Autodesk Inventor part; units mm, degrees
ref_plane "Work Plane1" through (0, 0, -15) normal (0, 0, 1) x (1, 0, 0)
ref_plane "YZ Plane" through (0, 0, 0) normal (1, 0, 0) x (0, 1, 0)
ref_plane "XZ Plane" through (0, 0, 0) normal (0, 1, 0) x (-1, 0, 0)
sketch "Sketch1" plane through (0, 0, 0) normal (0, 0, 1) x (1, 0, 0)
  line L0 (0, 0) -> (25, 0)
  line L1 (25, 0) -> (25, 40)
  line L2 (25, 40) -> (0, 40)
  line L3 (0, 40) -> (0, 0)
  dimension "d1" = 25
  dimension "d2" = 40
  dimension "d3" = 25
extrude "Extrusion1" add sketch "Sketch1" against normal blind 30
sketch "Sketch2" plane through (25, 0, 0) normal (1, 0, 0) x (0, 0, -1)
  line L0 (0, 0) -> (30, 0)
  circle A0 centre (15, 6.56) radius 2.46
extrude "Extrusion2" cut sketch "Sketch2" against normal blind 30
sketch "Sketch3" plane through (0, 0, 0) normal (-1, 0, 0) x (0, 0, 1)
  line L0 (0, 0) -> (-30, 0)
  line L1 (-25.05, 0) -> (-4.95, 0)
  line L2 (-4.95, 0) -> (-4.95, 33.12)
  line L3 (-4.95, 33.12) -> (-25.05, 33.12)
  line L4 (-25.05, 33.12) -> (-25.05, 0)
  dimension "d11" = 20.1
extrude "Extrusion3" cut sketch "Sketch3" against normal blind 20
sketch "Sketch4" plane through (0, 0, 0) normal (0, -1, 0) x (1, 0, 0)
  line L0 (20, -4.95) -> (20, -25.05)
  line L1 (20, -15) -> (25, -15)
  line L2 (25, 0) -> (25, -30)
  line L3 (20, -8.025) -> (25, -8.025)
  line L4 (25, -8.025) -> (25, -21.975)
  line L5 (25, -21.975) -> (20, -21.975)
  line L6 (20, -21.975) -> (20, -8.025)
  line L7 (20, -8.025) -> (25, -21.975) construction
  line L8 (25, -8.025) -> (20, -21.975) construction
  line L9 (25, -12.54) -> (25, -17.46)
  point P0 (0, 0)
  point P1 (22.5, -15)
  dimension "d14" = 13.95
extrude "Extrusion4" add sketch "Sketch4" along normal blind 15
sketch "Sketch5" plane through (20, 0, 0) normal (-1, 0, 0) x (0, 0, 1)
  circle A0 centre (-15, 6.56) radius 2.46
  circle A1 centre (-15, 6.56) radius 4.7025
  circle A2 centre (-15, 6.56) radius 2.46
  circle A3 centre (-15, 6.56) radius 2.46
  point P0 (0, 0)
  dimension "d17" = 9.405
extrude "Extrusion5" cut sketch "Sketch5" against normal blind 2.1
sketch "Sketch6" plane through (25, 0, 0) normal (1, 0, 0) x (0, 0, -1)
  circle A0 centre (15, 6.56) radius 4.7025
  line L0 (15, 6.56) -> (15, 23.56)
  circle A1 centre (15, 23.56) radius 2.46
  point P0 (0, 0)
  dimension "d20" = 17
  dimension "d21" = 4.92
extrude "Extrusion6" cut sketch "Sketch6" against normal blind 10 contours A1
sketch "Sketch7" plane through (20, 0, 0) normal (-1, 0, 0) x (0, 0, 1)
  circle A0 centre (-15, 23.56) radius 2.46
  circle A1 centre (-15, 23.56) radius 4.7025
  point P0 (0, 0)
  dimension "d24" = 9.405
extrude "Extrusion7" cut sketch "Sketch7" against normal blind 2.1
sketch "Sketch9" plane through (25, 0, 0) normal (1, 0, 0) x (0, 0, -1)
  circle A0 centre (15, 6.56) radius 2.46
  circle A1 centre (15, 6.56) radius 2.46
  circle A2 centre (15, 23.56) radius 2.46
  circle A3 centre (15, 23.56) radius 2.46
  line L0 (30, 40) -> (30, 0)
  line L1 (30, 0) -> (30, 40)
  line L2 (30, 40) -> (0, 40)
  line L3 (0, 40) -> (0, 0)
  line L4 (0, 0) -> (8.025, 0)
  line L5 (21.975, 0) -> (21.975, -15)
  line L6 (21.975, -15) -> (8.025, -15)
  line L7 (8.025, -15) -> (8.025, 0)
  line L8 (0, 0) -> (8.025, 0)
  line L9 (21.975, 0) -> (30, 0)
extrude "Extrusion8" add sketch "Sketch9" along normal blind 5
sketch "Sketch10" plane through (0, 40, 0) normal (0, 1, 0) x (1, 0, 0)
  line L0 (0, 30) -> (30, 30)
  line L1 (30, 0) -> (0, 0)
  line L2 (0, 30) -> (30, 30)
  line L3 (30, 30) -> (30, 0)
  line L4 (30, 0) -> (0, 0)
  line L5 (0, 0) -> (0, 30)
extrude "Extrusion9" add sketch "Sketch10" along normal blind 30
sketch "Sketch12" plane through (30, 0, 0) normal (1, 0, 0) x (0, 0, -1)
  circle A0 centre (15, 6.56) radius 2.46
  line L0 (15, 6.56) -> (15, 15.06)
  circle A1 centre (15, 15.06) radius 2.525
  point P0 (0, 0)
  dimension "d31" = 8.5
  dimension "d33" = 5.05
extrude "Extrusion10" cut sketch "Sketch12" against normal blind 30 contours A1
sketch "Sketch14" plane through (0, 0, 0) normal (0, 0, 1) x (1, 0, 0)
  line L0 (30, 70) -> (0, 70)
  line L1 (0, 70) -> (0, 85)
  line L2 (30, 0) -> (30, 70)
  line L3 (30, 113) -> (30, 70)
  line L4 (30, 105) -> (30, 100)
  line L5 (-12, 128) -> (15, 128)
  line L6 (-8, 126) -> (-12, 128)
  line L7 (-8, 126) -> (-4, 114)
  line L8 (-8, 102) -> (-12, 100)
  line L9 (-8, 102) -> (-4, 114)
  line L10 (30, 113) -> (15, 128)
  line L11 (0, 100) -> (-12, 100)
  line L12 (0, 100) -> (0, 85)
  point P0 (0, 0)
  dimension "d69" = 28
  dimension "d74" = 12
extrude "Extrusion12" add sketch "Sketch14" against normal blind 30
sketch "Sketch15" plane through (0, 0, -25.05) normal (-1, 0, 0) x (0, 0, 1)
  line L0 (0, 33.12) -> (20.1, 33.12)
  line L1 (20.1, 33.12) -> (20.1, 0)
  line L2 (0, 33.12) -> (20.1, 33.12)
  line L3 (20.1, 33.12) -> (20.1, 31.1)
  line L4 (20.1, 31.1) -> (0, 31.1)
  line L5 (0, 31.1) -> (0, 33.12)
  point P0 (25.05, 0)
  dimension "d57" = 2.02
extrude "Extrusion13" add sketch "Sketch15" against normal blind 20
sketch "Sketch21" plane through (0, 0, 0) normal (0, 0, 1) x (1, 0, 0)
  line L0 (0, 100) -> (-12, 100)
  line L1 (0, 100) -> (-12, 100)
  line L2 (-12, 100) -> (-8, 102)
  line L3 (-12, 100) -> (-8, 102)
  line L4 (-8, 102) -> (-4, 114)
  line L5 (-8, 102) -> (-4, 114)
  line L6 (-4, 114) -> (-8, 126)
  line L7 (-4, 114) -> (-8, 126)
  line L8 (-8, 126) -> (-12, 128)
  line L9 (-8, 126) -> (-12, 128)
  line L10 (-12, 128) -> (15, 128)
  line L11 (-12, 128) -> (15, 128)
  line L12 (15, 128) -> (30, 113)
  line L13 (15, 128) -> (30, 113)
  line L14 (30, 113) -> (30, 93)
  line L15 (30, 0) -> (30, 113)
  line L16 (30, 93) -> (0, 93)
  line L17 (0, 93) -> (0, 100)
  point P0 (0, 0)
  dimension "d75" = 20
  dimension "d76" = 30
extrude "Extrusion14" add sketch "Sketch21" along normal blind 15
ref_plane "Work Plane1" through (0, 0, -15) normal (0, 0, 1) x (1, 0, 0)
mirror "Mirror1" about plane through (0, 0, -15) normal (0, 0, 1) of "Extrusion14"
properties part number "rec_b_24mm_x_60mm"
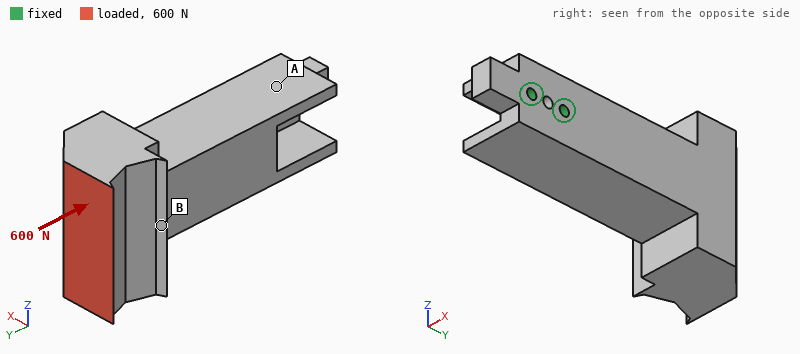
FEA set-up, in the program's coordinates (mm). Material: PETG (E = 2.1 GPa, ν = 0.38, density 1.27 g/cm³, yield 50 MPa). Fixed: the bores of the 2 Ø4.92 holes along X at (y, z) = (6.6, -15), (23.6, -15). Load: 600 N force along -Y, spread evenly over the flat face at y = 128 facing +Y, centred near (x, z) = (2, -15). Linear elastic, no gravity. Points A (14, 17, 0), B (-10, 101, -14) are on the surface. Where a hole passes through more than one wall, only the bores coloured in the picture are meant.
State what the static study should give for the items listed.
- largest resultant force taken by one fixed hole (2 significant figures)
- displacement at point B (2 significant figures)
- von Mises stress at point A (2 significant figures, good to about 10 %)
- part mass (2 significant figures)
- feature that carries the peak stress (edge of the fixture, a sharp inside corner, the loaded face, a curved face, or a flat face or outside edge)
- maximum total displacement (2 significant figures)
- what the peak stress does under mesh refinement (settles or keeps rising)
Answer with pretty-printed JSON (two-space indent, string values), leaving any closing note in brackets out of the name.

{
  "largest resultant force taken by one fixed hole": "670 N",
  "displacement at point B": "1.1 mm",
  "von Mises stress at point A": "4.3 MPa",
  "part mass": "180 g",
  "feature that carries the peak stress": "edge of the fixture",
  "maximum total displacement": "1.5 mm",
  "what the peak stress does under mesh refinement": "keeps rising"
}
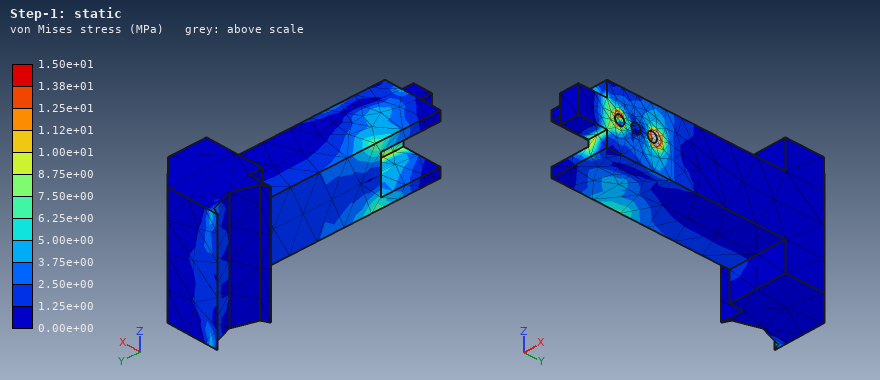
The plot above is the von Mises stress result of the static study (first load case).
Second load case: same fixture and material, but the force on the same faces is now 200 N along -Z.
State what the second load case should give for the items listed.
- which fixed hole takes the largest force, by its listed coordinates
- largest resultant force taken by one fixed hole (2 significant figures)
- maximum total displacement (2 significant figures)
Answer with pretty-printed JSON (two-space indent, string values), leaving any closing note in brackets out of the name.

{
  "which fixed hole takes the largest force, by its listed coordinates": "(23.6, -15)",
  "largest resultant force taken by one fixed hole": "1.1 kN",
  "maximum total displacement": "1.8 mm"
}
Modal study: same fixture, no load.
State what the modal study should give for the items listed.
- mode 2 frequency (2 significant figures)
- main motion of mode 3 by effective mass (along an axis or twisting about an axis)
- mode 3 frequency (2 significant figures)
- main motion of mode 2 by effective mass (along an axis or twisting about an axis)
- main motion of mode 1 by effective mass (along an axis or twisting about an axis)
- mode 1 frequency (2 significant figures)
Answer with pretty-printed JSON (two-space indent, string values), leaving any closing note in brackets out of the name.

{
  "mode 2 frequency": "220 Hz",
  "main motion of mode 3 by effective mass": "twisting about Y",
  "mode 3 frequency": "500 Hz",
  "main motion of mode 2 by effective mass": "along Z",
  "main motion of mode 1 by effective mass": "along X",
  "mode 1 frequency": "190 Hz"
}
